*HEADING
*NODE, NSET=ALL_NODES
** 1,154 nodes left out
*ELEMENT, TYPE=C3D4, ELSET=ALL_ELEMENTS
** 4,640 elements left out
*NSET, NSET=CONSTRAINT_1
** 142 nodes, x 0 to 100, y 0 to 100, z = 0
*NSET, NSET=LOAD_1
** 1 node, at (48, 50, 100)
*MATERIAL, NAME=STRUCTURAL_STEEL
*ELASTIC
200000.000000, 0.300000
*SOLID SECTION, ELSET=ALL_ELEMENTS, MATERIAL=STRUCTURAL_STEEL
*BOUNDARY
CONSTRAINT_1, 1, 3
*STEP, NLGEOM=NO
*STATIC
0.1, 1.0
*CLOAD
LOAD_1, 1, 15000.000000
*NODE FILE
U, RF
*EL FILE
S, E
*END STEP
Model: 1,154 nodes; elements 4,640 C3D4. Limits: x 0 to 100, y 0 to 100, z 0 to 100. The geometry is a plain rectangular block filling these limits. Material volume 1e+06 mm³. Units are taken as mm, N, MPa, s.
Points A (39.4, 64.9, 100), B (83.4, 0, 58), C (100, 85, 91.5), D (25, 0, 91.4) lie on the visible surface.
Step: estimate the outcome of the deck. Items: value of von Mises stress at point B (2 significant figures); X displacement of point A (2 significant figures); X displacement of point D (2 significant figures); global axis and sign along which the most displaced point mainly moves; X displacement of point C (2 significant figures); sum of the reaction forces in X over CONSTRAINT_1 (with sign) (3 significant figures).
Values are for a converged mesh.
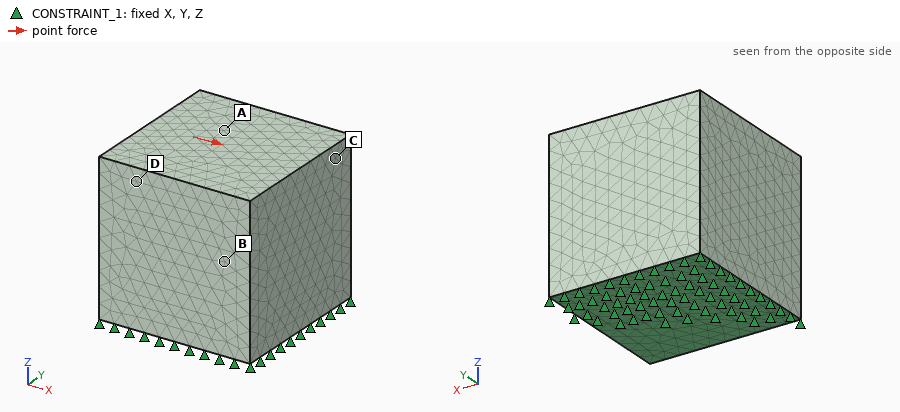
3.1 MPa
0.0055 mm
0.0040 mm
+X
0.0042 mm
-15000 N
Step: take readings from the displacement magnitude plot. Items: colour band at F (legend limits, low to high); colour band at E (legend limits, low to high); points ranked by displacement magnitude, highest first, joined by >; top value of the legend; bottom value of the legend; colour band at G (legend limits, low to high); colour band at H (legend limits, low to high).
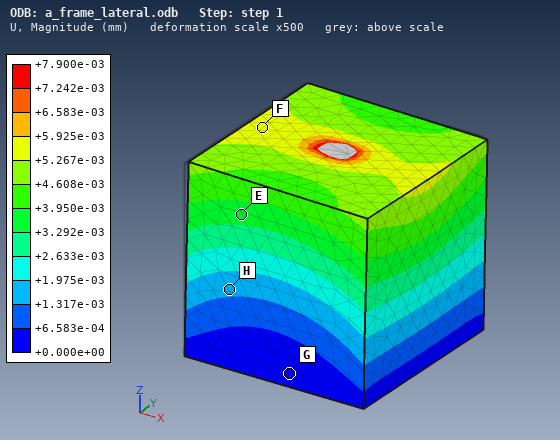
+5.267e-03 to +5.925e-03 mm
+3.292e-03 to +3.950e-03 mm
F > E > H > G
+7.900e-03 mm
+0.000e+00 mm
+0.000e+00 to +6.583e-04 mm
+1.317e-03 to +1.975e-03 mm
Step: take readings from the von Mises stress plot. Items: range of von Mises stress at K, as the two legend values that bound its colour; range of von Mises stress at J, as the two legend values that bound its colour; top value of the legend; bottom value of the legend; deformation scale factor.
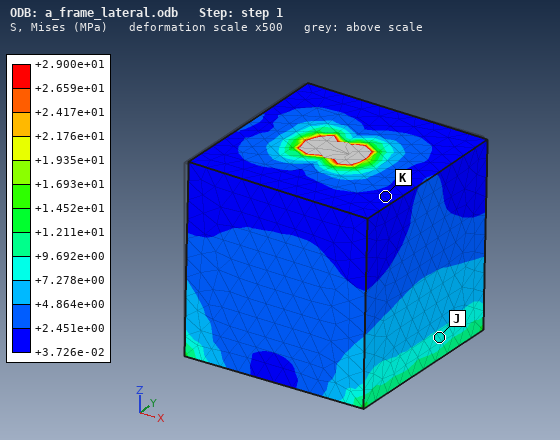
+3.726e-02 to +2.451e+00 MPa
+7.278e+00 to +9.692e+00 MPa
+2.900e+01 MPa
+3.726e-02 MPa
500
